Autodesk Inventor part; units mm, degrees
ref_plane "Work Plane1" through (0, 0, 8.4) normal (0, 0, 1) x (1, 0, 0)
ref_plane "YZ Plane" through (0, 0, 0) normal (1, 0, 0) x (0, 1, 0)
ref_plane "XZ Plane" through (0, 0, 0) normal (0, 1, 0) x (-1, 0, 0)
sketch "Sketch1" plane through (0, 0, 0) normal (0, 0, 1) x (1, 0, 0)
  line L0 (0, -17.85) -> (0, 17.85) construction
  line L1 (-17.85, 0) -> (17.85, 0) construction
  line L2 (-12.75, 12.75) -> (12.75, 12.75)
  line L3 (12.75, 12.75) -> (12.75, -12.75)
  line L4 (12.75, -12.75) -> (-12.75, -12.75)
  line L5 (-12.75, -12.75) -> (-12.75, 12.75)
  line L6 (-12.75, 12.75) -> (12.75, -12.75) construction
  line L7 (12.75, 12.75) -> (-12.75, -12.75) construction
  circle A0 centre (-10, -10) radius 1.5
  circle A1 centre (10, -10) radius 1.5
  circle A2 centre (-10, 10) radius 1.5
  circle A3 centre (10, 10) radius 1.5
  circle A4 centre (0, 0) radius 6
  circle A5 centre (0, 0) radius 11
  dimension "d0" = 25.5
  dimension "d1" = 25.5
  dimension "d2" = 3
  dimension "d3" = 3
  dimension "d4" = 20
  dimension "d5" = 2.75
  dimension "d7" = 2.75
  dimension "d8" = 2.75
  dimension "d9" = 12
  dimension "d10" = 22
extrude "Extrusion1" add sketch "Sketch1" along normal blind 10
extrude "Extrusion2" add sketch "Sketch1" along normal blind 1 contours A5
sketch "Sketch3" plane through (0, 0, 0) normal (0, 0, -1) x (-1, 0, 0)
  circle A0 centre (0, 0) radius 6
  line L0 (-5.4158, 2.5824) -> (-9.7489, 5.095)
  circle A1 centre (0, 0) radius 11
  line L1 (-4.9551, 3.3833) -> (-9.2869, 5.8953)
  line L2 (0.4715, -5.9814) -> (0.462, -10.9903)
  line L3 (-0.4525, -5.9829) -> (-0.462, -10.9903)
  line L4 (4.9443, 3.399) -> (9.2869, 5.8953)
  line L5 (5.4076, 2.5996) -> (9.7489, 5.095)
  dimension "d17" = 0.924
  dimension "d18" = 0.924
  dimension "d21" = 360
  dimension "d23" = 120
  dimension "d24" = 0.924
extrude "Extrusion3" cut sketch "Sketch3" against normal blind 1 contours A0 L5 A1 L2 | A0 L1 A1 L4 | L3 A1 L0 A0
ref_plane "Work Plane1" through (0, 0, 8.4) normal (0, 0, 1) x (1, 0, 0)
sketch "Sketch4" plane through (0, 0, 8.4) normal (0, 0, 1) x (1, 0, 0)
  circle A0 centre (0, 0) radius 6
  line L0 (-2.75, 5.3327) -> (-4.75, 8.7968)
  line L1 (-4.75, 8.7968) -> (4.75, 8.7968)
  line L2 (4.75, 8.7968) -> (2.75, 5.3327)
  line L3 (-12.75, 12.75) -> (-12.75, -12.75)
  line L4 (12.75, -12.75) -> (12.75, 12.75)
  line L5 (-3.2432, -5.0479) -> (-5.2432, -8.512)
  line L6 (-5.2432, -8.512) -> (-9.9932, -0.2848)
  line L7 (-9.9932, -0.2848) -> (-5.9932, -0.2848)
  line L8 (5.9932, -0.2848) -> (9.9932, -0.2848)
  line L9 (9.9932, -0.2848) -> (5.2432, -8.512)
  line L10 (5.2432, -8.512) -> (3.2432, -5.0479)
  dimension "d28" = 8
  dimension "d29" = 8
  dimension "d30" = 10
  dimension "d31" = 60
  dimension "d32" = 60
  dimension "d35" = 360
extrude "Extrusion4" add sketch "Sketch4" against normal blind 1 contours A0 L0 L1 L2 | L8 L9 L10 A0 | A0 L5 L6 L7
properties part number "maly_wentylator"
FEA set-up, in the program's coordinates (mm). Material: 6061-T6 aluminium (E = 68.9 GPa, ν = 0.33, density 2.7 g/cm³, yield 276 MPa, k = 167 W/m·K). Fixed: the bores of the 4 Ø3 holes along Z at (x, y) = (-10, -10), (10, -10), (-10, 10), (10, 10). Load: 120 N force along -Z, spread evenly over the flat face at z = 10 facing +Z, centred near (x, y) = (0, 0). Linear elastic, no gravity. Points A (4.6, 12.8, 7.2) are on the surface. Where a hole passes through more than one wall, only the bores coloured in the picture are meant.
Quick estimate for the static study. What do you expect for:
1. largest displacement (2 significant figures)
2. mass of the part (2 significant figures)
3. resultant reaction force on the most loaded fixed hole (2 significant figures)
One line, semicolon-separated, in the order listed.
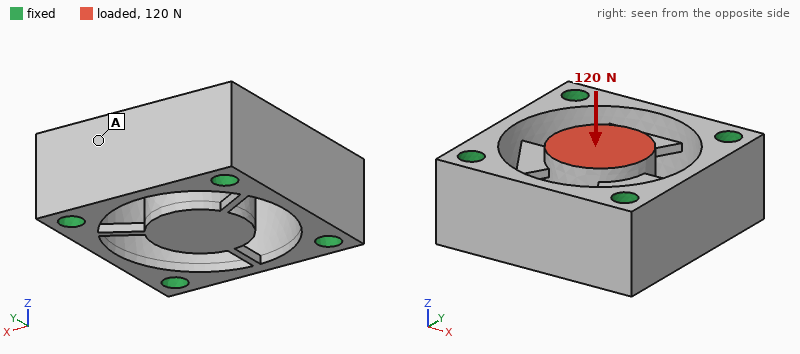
0.12 mm; 9.8 g; 36 N
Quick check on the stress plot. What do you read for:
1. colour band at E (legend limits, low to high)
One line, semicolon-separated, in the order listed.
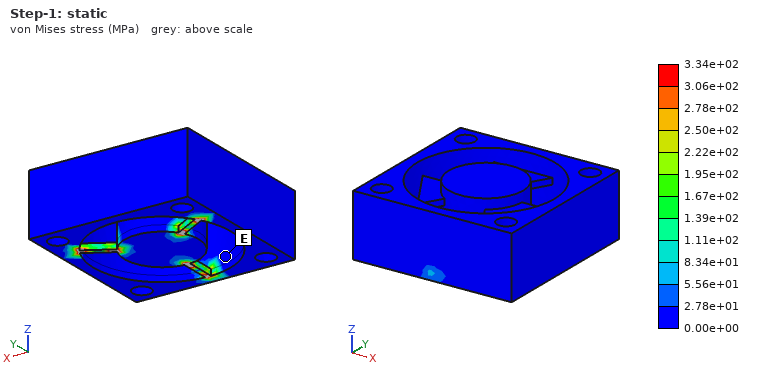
0.00e+00 to 2.78e+01 MPa
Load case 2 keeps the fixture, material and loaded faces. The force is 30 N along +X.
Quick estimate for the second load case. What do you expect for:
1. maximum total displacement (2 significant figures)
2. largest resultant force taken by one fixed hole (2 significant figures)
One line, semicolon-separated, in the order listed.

93 µm; 22 N
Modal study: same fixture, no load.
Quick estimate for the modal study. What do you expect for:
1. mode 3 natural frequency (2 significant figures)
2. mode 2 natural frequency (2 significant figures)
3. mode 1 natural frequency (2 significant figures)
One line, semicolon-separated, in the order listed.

2800 Hz; 2700 Hz; 2700 Hz
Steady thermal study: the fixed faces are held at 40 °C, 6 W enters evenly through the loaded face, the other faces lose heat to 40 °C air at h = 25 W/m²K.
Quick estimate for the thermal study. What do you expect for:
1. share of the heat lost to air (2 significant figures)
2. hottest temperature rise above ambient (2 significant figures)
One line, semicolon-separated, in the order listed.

19 %; 66 K
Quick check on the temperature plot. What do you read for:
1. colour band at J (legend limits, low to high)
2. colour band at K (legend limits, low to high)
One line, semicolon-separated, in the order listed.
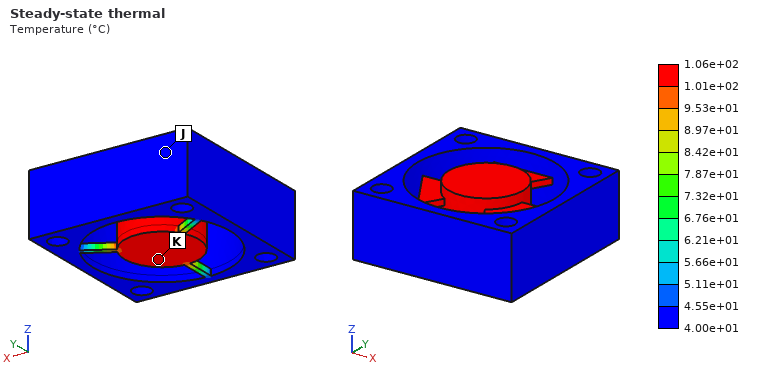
4.00e+01 to 4.55e+01 °C; 1.01e+02 to 1.06e+02 °C
